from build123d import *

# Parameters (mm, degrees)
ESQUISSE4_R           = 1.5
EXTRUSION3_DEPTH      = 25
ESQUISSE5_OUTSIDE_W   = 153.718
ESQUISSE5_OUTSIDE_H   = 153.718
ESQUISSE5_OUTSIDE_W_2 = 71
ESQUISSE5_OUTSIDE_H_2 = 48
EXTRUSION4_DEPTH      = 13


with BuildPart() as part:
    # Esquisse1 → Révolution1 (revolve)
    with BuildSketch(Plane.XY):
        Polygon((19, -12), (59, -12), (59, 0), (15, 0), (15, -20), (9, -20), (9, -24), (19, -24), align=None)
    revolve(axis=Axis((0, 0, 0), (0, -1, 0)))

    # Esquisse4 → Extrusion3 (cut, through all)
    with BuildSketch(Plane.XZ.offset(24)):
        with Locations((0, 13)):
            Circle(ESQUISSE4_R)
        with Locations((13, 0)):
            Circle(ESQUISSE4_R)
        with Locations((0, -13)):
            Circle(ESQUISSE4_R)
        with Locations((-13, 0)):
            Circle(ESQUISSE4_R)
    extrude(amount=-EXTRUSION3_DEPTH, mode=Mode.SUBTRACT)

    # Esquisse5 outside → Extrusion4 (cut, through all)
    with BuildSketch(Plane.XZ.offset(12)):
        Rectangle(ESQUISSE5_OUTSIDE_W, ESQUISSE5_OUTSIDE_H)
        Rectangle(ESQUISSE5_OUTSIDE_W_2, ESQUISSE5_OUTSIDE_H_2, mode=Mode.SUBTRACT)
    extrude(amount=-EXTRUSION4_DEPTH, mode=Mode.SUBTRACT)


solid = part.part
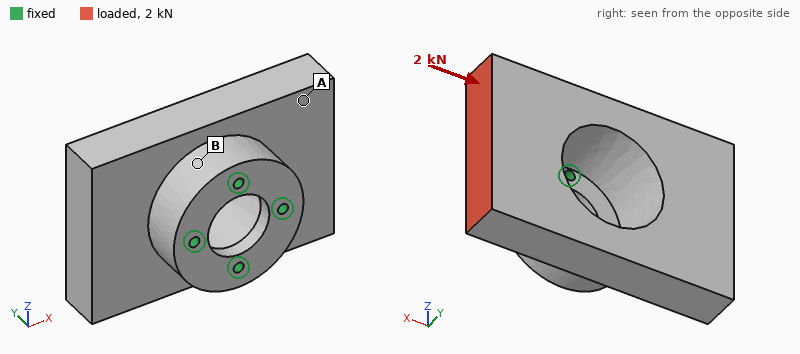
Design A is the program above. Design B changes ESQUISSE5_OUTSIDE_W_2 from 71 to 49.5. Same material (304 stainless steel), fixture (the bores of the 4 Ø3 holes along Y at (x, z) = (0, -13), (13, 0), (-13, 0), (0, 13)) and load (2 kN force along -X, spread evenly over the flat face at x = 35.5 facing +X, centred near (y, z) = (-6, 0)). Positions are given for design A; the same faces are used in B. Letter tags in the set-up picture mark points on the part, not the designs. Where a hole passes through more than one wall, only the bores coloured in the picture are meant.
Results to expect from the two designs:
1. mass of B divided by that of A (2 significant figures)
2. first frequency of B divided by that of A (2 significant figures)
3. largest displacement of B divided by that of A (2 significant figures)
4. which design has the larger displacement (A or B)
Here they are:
0.68
1.5
0.92
A
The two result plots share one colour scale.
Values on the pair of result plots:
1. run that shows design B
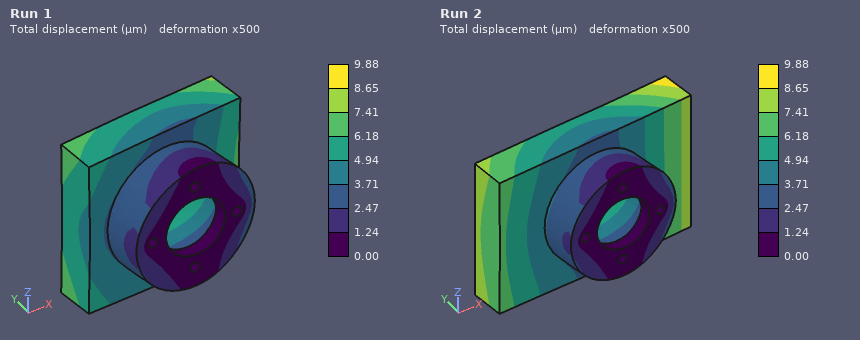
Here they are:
Run 1
